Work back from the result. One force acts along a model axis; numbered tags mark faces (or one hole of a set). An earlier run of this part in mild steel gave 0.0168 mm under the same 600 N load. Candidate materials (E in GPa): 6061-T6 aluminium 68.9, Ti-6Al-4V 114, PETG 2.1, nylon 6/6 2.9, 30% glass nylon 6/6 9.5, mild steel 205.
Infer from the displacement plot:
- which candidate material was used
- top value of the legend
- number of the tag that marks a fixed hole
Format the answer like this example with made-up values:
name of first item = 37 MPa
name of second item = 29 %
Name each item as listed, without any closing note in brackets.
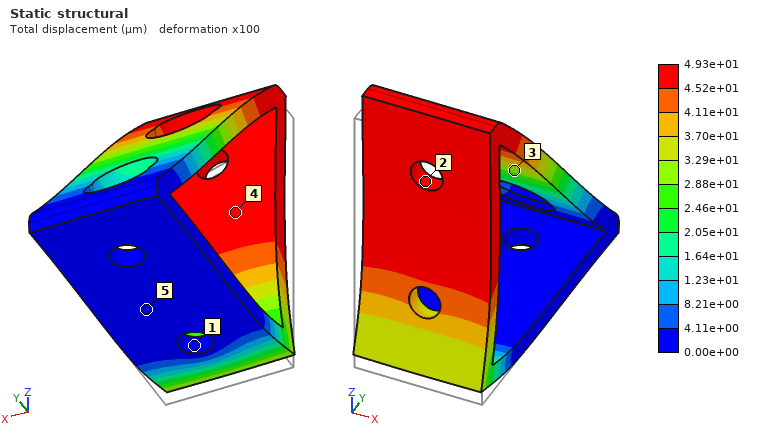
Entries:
which candidate material was used = 6061-T6 aluminium
top value of the legend = 4.93e+01 µm
number of the tag that marks a fixed hole = 1
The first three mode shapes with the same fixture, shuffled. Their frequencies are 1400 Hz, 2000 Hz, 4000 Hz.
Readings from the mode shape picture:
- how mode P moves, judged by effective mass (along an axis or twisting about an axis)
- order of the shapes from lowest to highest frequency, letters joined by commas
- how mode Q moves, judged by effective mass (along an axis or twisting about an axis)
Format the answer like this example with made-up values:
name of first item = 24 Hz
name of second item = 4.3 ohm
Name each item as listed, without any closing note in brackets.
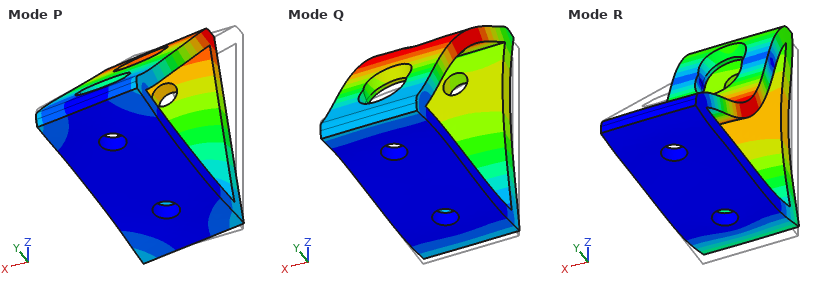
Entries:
how mode P moves, judged by effective mass = along X
order of the shapes from lowest to highest frequency, letters joined by commas = P, Q, R
how mode Q moves, judged by effective mass = along Y
